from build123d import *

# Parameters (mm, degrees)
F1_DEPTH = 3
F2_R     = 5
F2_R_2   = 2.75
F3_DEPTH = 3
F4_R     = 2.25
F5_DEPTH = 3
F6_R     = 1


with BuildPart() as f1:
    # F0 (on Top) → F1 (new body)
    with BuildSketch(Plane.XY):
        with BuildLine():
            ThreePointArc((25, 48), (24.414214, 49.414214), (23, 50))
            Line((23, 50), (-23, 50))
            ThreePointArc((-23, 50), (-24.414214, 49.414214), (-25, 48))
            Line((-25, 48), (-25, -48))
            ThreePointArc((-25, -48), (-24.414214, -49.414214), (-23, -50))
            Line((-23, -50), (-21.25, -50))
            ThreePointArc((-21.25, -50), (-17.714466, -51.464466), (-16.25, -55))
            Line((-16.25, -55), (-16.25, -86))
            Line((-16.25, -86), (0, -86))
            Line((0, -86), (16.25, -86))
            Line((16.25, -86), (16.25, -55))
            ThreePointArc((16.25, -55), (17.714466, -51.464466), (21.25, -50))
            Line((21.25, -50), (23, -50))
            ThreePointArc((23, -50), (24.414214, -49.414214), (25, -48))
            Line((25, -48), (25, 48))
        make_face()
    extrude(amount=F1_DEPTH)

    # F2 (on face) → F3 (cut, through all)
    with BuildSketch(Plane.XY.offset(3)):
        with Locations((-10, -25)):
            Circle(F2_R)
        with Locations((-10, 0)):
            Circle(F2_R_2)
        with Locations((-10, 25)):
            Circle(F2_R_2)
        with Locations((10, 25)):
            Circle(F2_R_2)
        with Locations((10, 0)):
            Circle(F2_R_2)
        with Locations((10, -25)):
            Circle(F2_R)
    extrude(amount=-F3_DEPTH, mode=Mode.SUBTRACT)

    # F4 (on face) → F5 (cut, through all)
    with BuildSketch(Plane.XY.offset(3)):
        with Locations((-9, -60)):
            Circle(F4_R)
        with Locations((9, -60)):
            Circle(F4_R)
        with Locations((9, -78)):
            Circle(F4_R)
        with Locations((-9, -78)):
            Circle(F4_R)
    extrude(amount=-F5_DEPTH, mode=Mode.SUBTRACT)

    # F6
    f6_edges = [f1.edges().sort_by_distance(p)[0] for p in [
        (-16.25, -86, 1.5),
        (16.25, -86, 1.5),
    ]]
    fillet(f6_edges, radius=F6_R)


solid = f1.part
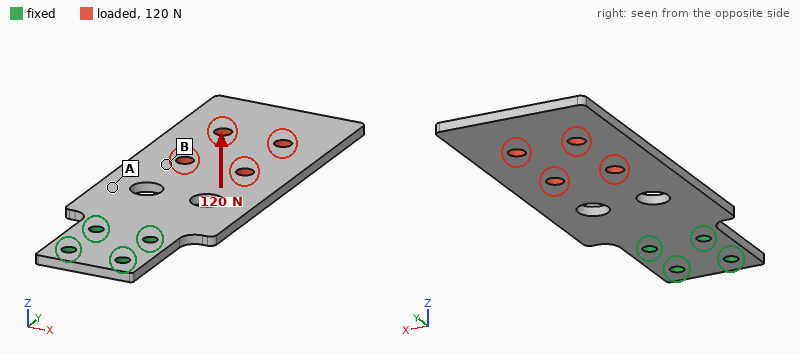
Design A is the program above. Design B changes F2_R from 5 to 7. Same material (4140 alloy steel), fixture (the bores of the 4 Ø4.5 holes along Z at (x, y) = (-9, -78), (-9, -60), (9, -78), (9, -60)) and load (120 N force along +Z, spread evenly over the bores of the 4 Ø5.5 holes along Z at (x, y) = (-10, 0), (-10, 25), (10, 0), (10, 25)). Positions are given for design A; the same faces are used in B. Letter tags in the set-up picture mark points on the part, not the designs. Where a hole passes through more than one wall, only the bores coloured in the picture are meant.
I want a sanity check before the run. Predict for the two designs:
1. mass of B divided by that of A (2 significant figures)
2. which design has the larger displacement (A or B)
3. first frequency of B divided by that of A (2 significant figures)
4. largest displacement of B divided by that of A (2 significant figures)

0.97
B
0.96
1.1
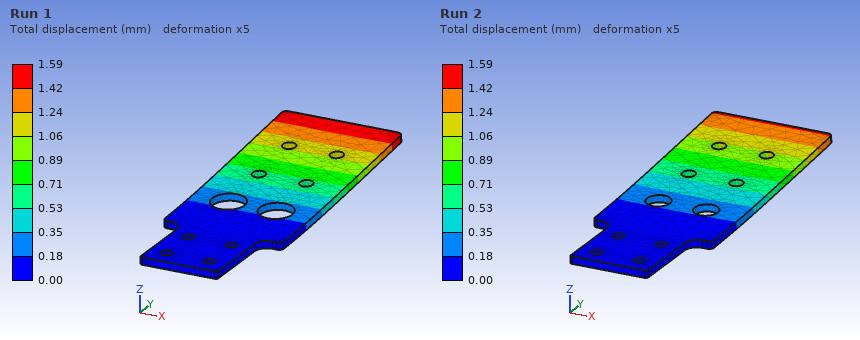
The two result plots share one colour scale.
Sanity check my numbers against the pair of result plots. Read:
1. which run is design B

Run 1
